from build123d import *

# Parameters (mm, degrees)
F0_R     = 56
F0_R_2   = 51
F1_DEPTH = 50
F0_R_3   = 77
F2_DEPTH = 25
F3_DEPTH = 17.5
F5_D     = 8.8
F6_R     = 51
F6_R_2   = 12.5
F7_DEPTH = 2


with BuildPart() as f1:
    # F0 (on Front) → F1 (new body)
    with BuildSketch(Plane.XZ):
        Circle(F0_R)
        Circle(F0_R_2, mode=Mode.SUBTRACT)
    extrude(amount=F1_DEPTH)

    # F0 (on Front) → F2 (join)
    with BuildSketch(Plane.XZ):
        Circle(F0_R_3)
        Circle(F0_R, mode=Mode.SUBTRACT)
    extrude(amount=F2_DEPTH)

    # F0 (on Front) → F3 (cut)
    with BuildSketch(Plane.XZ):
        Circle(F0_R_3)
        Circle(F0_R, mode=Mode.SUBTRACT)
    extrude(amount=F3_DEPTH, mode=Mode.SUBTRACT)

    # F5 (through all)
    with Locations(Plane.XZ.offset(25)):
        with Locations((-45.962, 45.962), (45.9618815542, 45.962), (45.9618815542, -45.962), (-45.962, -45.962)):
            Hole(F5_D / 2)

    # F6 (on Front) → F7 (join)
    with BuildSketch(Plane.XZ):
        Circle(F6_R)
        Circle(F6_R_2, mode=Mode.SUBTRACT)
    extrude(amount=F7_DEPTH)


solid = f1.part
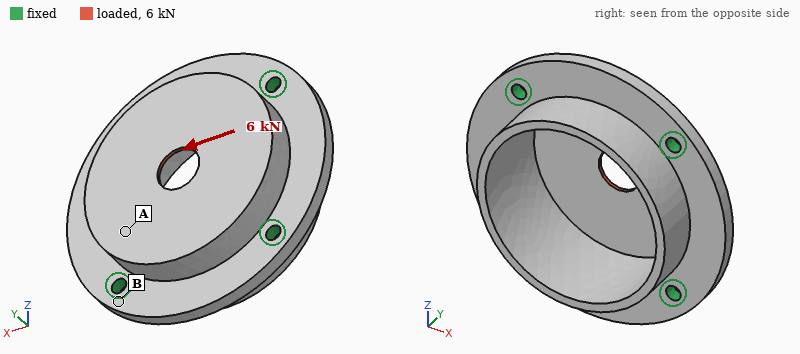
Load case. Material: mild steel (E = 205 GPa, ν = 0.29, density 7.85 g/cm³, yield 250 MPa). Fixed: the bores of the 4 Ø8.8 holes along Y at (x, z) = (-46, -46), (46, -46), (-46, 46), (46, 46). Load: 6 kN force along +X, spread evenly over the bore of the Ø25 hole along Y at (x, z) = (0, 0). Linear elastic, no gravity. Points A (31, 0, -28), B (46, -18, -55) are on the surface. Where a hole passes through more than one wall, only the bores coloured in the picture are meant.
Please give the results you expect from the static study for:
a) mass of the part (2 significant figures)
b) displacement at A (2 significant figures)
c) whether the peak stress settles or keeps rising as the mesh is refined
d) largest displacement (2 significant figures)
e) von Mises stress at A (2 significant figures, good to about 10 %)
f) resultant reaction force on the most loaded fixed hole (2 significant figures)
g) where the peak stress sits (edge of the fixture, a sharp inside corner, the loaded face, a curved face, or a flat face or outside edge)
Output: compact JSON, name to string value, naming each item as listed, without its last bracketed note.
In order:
{"mass of the part": "1.3 kg", "displacement at A": "8.9 µm", "whether the peak stress settles or keeps rising as the mesh is refined": "keeps rising", "largest displacement": "14 µm", "von Mises stress at A": "22 MPa", "resultant reaction force on the most loaded fixed hole": "1.7 kN", "where the peak stress sits": "a sharp inside corner"}
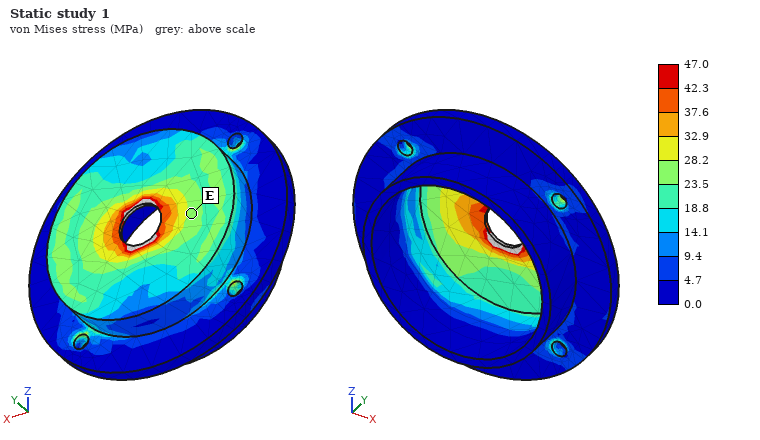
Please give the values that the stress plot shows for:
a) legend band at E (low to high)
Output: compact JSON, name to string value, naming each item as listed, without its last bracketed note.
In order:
{"legend band at E": "23.5 to 28.2 MPa"}
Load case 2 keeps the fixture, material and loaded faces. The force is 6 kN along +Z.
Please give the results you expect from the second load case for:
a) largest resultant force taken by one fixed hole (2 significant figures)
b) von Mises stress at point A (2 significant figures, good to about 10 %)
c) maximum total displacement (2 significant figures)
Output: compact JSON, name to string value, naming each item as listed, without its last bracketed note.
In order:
{"largest resultant force taken by one fixed hole": "1.7 kN", "von Mises stress at point A": "21 MPa", "maximum total displacement": "14 µm"}
